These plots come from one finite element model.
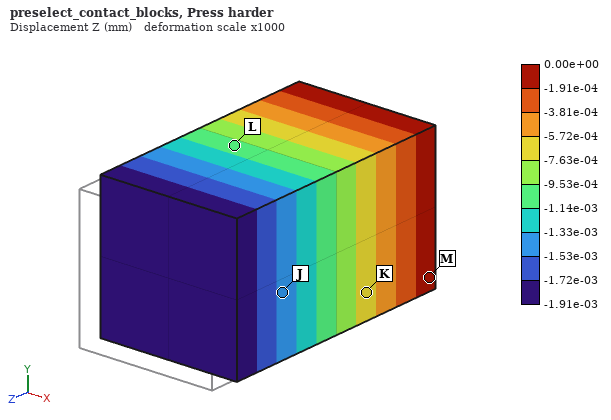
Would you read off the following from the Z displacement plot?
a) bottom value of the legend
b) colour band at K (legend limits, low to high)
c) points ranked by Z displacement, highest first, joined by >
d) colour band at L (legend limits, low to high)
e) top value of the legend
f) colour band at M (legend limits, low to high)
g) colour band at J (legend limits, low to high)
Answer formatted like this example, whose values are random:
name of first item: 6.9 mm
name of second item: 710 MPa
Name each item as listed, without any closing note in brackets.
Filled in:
bottom value of the legend: -1.91e-03 mm
colour band at K: -7.63e-04 to -5.72e-04 mm
points ranked by Z displacement, highest first, joined by >: M > K > L > J
colour band at L: -1.14e-03 to -9.53e-04 mm
top value of the legend: 0.00e+00 mm
colour band at M: -1.91e-04 to 0.00e+00 mm
colour band at J: -1.53e-03 to -1.33e-03 mm
